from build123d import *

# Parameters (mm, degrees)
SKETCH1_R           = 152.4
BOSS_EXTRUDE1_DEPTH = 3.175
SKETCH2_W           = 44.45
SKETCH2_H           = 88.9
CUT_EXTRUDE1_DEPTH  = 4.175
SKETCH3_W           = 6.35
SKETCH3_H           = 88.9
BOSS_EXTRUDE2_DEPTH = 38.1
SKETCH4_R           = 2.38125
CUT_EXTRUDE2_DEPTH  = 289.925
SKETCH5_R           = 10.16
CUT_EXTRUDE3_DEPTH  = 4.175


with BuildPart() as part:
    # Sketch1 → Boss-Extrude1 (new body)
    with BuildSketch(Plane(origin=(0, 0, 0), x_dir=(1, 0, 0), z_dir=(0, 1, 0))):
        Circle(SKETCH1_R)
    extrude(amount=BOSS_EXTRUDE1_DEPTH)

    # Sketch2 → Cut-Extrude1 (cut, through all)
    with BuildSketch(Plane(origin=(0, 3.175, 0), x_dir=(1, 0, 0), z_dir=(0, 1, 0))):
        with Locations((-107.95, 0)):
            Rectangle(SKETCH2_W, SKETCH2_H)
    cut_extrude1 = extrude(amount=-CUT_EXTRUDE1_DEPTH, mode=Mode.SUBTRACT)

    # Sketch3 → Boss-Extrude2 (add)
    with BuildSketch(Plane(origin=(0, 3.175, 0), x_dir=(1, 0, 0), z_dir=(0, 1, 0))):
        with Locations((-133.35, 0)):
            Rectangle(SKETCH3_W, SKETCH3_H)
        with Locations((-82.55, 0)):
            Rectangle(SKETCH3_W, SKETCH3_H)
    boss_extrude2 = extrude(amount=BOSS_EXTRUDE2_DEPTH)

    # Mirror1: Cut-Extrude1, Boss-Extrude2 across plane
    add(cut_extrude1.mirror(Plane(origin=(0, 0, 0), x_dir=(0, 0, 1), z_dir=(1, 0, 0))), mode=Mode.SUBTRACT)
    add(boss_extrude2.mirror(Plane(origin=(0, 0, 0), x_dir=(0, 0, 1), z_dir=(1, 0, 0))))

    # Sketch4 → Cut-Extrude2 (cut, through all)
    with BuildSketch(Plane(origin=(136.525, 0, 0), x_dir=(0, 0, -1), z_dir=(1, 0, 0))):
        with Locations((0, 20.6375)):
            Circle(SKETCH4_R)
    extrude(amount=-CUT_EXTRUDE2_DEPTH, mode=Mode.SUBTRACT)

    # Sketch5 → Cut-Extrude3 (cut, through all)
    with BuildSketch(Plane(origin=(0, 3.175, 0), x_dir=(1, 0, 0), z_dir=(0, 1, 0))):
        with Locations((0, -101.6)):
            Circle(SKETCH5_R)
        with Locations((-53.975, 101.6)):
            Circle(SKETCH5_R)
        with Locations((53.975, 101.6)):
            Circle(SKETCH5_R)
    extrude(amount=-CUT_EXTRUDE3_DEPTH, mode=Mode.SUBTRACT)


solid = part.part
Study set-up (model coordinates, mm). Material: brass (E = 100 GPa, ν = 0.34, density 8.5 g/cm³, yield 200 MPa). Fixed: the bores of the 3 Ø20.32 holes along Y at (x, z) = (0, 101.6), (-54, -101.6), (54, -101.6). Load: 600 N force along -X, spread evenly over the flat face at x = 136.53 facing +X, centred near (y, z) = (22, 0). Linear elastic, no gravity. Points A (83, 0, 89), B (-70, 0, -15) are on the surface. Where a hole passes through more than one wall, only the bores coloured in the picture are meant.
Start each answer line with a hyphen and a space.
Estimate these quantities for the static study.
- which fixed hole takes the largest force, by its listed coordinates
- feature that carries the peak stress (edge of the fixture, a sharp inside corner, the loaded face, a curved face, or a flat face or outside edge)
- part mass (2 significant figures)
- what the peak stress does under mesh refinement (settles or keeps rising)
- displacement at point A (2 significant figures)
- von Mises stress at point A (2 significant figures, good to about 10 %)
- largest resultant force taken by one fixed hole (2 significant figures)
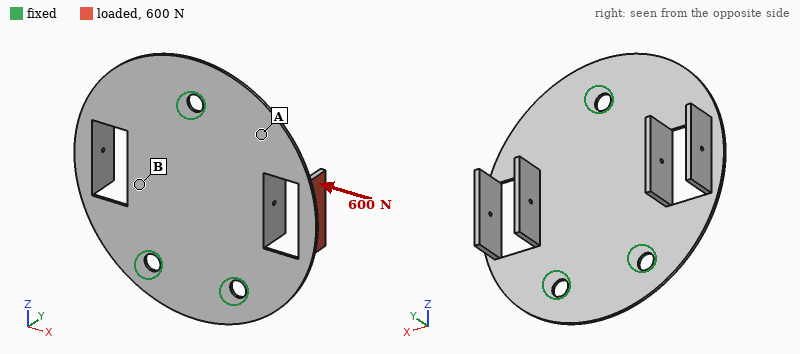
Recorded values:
- (0, 101.6)
- a sharp inside corner
- 2.5 kg
- keeps rising
- 0.42 mm
- 34 MPa
- 340 N
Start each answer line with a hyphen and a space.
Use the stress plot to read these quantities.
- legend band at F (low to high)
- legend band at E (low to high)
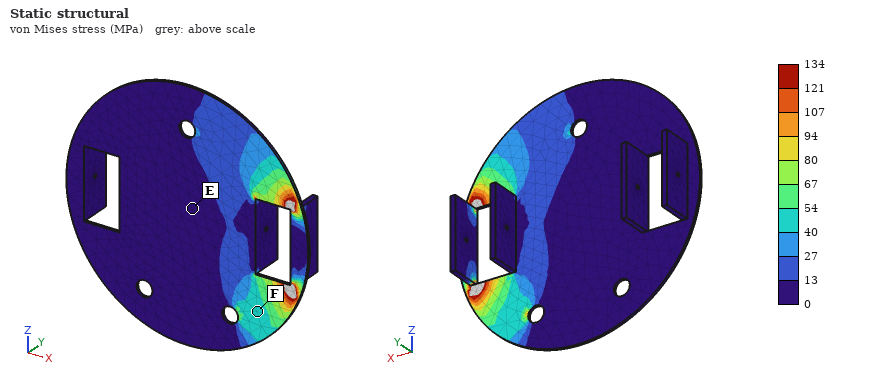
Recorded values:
- 40 to 54 MPa
- 0 to 13 MPa
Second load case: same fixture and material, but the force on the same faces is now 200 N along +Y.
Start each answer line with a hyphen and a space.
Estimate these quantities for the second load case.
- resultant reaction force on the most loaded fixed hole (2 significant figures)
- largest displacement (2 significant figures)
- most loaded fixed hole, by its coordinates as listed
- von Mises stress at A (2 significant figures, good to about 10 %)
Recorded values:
- 160 N
- 2.1 mm
- (54, -101.6)
- 26 MPa
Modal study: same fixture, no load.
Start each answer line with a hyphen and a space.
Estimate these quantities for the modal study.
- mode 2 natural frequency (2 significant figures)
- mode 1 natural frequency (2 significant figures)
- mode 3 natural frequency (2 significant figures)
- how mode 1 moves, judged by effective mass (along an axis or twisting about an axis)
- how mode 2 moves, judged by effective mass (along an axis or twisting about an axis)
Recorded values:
- 97 Hz
- 92 Hz
- 230 Hz
- twisting about Z
- along Y
